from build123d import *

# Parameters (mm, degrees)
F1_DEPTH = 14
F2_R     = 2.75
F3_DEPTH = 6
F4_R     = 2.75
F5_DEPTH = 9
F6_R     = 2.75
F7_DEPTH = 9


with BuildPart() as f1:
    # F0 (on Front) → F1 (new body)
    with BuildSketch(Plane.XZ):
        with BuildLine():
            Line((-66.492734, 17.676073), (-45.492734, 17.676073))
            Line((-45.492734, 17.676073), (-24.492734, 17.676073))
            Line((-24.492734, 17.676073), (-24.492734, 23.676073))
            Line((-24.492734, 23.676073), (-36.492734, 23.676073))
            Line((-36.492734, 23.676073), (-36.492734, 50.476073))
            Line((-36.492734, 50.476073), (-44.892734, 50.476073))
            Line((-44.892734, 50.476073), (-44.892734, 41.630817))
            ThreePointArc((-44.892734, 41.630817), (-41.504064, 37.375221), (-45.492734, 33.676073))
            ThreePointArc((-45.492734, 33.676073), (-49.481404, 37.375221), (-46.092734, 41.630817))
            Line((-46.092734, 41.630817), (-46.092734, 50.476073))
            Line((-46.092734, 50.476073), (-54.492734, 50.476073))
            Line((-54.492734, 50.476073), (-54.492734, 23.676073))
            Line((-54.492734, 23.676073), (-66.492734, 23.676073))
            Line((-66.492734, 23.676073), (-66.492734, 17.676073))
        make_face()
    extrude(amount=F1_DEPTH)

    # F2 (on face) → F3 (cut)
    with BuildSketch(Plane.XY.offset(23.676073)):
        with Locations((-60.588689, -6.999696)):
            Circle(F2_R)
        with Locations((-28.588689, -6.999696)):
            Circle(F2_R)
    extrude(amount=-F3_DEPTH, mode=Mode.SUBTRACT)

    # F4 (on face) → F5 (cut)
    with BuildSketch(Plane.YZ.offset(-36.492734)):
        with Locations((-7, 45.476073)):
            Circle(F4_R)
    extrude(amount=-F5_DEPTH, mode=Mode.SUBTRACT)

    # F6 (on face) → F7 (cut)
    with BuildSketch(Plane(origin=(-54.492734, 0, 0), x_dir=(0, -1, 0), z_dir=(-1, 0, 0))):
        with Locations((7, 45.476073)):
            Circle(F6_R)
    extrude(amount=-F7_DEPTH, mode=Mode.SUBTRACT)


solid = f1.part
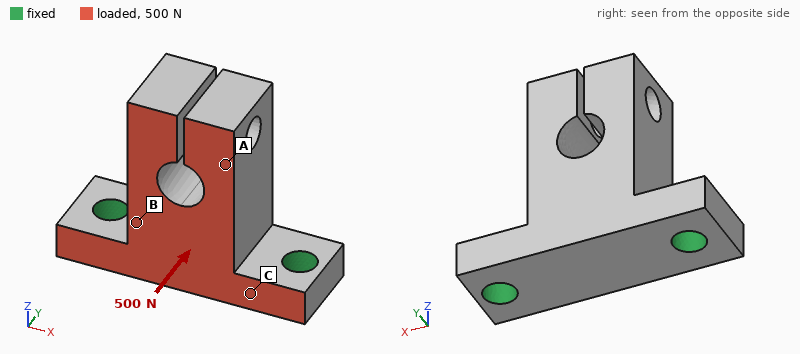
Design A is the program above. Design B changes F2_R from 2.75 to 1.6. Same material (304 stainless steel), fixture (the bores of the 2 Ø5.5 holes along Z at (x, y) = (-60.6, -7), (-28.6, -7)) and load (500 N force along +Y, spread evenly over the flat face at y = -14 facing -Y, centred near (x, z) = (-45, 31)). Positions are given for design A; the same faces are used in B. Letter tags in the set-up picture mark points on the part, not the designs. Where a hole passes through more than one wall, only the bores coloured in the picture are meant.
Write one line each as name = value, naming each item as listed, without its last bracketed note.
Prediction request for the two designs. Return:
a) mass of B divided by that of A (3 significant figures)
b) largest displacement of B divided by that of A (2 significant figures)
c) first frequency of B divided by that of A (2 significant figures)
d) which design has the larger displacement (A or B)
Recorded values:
mass of B divided by that of A = 1.02
largest displacement of B divided by that of A = 1.3
first frequency of B divided by that of A = 0.87
which design has the larger displacement = B
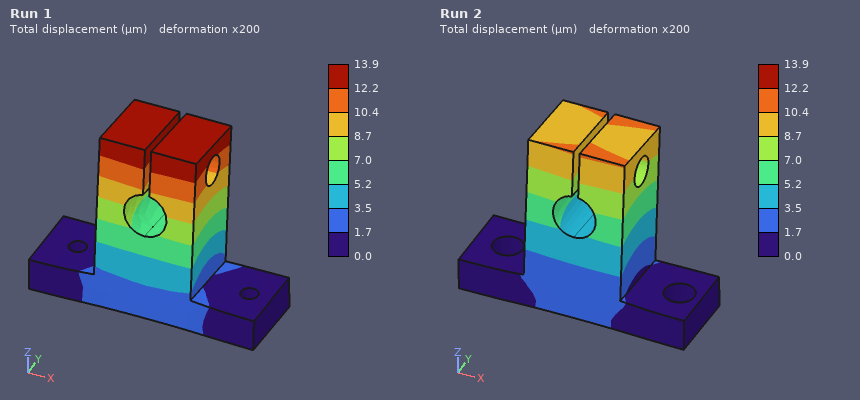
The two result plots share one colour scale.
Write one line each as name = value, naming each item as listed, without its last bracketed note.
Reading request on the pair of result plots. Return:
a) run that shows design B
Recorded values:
run that shows design B = Run 1
